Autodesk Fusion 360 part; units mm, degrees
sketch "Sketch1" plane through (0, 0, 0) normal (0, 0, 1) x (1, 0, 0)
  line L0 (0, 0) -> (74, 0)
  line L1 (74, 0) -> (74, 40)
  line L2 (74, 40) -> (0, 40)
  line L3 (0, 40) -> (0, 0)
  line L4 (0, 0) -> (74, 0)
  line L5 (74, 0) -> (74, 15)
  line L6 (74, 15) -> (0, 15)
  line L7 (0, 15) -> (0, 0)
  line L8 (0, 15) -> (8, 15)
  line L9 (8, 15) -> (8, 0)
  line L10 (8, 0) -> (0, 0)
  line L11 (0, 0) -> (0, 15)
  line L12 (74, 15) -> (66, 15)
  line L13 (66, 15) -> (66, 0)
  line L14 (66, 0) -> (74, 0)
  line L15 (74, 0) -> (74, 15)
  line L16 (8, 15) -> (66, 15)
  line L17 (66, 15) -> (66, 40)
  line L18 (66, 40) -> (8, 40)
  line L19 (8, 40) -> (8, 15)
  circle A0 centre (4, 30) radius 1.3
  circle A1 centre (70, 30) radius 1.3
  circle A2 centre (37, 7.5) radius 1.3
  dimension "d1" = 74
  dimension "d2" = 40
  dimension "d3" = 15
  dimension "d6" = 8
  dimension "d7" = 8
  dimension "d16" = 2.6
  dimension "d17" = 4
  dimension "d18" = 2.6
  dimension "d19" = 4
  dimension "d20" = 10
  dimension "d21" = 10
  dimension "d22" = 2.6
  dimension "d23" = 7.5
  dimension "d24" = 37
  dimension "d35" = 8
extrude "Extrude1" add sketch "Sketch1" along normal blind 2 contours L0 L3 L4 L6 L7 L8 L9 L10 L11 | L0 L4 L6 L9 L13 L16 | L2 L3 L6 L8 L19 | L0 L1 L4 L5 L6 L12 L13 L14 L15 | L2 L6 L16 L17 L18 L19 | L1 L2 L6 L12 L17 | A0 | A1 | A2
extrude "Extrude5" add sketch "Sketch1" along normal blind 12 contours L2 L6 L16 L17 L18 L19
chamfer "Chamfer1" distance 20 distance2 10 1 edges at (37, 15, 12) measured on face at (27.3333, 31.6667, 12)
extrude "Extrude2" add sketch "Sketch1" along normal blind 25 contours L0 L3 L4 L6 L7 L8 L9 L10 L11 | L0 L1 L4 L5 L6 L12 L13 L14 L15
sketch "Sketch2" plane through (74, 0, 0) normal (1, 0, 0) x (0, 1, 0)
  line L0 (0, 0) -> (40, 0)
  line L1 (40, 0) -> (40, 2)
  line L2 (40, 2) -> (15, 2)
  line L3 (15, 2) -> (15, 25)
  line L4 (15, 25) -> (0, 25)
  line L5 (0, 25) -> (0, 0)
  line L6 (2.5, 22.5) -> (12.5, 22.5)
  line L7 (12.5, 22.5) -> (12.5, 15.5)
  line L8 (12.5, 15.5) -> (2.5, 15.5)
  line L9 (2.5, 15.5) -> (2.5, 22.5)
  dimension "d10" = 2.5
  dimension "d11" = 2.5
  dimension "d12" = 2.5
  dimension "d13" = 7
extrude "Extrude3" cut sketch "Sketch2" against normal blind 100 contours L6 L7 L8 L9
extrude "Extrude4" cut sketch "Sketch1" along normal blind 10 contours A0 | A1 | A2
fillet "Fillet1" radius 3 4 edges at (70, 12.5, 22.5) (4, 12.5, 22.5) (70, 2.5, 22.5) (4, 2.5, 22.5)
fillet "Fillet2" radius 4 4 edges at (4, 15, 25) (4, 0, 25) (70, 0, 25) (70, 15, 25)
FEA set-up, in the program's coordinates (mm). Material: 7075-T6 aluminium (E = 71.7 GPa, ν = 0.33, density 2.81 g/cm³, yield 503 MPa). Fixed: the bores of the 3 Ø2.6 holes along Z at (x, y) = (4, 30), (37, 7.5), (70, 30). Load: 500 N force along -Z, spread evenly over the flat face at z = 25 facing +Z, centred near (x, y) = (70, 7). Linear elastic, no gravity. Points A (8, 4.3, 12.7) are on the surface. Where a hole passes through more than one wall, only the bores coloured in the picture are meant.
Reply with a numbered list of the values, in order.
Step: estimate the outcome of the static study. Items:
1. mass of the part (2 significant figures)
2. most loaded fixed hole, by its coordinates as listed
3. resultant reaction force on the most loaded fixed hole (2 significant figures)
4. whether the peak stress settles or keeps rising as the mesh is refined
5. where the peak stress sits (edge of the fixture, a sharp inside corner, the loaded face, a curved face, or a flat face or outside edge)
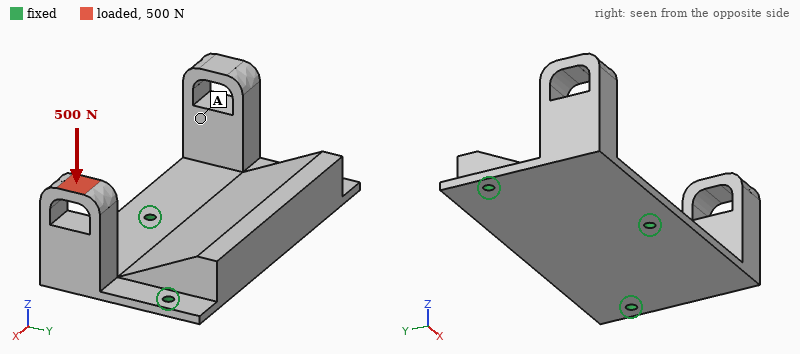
1. 53 g
2. (37, 7.5)
3. 680 N
4. keeps rising
5. a sharp inside corner
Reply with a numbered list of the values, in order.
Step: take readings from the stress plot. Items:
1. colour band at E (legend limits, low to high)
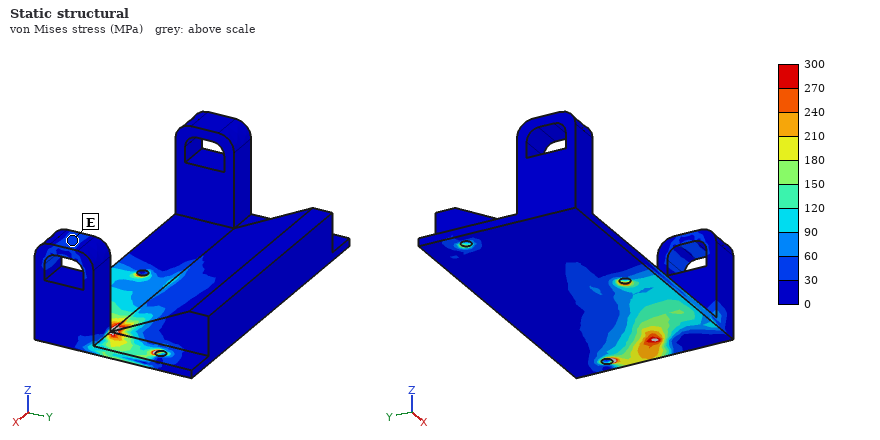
1. 30 to 60 MPa
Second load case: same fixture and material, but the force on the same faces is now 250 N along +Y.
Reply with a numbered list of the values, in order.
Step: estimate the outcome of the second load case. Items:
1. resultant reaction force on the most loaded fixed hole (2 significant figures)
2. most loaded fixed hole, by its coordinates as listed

1. 370 N
2. (37, 7.5)
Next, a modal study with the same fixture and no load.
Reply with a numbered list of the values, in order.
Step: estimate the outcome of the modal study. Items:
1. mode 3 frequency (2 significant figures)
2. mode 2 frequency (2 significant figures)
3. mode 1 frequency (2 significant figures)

1. 2600 Hz
2. 1500 Hz
3. 1400 Hz
